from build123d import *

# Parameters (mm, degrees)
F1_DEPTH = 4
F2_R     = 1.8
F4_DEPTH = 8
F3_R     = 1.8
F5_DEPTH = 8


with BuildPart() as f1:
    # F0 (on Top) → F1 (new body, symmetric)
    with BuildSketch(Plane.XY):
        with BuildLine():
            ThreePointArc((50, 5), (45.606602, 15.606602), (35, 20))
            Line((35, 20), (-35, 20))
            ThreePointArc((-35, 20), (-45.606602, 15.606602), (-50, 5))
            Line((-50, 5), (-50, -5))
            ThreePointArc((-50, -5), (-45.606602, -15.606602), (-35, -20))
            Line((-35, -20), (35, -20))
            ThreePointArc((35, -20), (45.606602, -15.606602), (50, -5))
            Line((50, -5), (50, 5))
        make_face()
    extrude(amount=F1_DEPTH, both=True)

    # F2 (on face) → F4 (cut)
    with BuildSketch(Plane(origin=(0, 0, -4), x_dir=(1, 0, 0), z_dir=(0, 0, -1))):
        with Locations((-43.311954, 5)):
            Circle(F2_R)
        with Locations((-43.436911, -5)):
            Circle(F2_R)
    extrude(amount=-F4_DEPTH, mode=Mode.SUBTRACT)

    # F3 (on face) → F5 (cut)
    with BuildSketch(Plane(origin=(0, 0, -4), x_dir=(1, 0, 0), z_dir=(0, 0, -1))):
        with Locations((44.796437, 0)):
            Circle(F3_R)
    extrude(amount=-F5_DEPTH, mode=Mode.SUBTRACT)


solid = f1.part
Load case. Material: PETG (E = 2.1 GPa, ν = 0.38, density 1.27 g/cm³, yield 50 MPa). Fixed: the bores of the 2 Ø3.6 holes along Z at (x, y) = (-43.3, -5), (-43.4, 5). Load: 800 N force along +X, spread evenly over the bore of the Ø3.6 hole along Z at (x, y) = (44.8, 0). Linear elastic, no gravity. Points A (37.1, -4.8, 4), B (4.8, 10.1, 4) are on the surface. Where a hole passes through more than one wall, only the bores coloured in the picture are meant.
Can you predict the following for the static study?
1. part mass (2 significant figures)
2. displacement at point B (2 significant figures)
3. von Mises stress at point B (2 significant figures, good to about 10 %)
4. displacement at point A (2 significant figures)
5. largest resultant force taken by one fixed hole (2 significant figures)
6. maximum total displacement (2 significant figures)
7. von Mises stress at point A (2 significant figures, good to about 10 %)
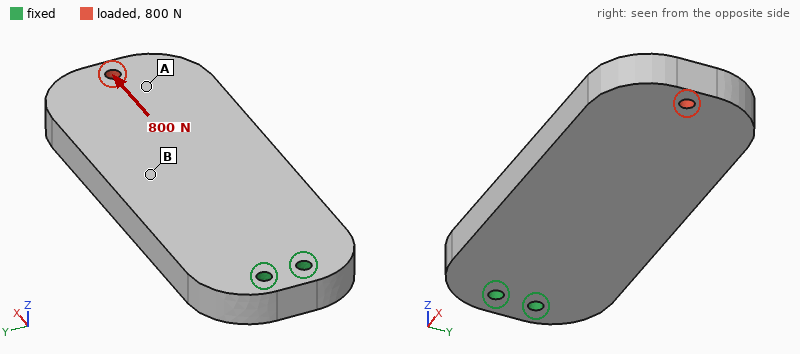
38 g
0.071 mm
2.5 MPa
0.12 mm
400 N
0.17 mm
5.2 MPa
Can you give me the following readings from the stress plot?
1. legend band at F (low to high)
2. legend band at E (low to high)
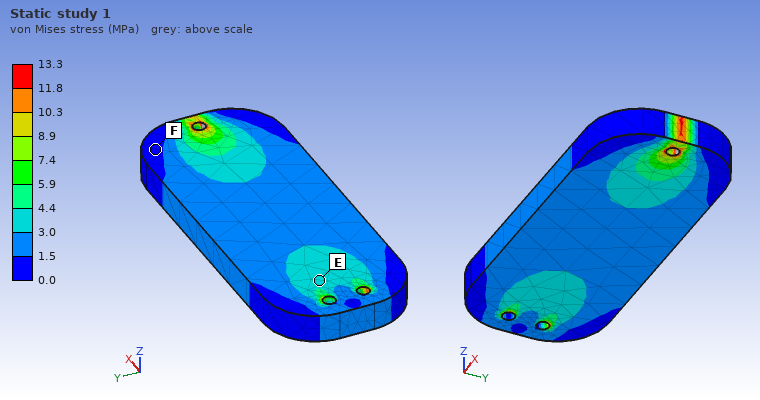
0.0 to 1.5 MPa
3.0 to 4.4 MPa
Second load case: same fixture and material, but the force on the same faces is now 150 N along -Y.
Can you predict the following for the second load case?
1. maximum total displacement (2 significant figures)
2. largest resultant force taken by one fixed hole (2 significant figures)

1.2 mm
1.0 kN
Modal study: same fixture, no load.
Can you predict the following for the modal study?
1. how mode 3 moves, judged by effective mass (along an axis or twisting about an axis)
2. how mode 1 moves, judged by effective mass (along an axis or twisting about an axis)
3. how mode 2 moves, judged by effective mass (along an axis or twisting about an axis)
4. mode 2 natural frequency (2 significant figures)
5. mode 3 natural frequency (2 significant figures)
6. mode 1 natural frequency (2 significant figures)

twisting about X
along Z
along Y
530 Hz
830 Hz
190 Hz
